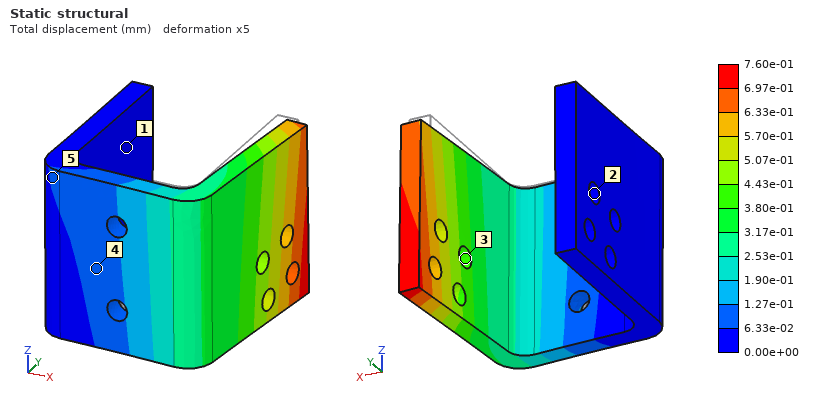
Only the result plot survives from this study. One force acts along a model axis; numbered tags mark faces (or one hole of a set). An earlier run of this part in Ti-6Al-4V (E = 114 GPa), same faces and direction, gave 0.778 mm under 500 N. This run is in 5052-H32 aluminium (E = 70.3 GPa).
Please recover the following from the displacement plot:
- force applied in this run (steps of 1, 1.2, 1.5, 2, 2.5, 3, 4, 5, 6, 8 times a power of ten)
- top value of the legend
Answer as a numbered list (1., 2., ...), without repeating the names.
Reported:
1. 300 N
2. 7.60e-01 mm
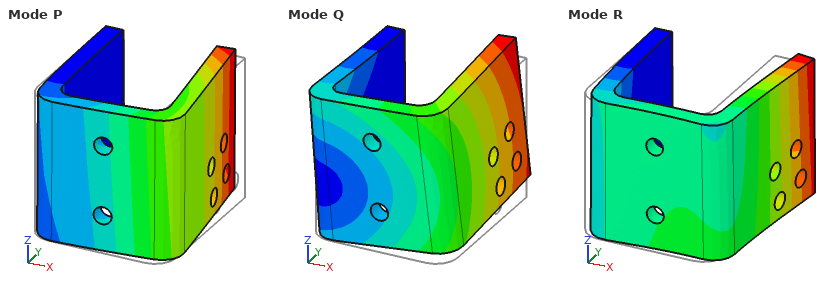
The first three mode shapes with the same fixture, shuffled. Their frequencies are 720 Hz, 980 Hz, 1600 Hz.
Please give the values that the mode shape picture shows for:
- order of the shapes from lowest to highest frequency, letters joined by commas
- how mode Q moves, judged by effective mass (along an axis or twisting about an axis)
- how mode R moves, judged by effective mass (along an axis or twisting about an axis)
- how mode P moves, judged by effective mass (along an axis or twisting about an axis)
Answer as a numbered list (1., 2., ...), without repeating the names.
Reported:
1. P, Q, R
2. along Z
3. along X
4. along Y
